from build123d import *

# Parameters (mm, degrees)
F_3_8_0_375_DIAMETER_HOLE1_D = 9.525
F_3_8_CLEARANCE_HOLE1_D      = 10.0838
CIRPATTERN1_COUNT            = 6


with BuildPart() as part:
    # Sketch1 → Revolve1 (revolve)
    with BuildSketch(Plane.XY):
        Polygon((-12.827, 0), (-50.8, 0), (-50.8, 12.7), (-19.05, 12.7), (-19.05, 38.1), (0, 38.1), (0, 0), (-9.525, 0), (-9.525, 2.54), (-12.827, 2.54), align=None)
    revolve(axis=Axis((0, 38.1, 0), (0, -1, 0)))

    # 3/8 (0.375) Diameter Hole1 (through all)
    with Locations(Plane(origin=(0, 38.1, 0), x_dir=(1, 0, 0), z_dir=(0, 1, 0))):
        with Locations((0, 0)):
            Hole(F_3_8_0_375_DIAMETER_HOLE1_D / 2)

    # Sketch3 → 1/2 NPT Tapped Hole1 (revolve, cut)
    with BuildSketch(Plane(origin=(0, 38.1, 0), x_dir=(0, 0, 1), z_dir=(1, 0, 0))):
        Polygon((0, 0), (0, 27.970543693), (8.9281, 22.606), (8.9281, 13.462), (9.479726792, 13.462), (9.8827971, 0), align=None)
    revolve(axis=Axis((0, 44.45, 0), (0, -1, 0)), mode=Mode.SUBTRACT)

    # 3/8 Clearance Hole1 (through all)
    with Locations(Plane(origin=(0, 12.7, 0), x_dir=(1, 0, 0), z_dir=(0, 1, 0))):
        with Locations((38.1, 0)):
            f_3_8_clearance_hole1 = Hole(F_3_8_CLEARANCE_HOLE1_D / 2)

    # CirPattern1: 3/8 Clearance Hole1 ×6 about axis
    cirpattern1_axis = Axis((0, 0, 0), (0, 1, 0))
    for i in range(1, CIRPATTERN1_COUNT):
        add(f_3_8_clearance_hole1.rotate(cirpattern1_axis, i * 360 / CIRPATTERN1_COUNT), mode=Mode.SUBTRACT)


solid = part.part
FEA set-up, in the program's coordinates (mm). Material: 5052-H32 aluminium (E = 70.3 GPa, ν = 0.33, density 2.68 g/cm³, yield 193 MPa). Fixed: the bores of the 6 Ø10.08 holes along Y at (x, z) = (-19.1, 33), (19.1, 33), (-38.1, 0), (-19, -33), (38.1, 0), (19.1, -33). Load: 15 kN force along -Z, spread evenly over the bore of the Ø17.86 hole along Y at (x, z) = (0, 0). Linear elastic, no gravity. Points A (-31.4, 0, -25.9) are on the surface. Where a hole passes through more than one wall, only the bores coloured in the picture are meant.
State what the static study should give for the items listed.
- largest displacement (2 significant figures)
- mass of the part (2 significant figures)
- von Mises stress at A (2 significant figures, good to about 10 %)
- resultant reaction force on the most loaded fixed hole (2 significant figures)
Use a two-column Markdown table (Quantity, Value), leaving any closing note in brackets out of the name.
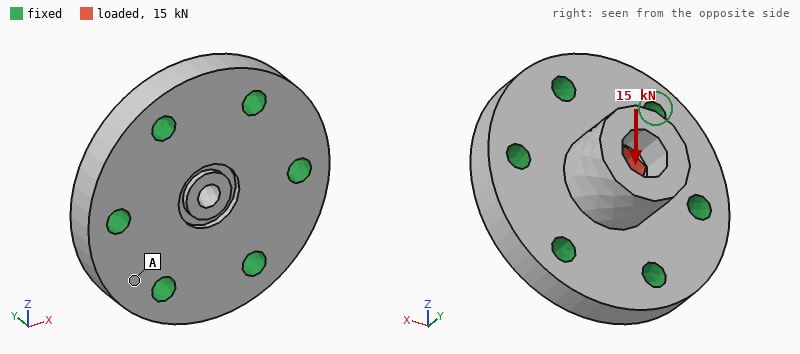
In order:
| Quantity | Value |
|---|---|
| largest displacement | 24 µm |
| mass of the part | 320 g |
| von Mises stress at A | 4.7 MPa |
| resultant reaction force on the most loaded fixed hole | 4.0 kN |
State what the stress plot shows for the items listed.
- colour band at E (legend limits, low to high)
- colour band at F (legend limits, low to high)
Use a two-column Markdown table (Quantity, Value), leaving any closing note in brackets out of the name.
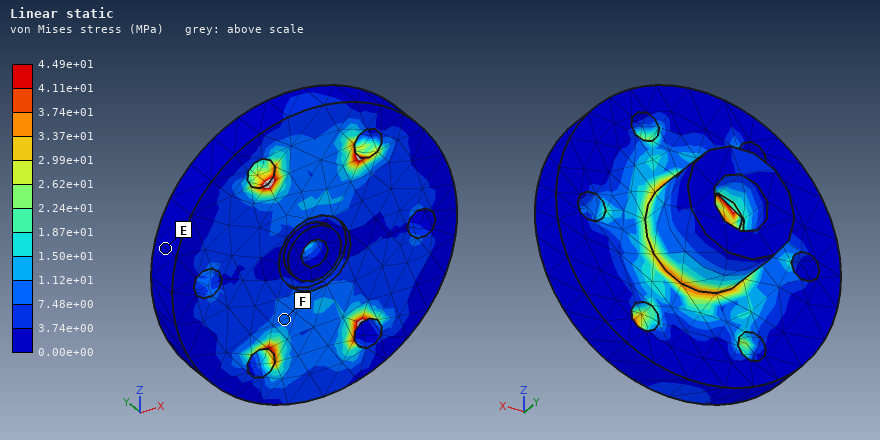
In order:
| Quantity | Value |
|---|---|
| colour band at E | 0.00e+00 to 3.74e+00 MPa |
| colour band at F | 7.48e+00 to 1.12e+01 MPa |
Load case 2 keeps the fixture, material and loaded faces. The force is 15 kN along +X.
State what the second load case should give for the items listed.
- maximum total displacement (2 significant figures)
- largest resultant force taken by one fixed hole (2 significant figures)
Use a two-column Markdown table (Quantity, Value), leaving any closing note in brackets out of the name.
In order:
| Quantity | Value |
|---|---|
| maximum total displacement | 24 µm |
| largest resultant force taken by one fixed hole | 4.5 kN |
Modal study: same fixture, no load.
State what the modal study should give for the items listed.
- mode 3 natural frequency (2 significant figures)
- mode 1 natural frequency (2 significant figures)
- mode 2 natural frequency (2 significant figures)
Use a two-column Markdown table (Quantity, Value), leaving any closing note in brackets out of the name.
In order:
| Quantity | Value |
|---|---|
| mode 3 natural frequency | 14 kHz |
| mode 1 natural frequency | 14 kHz |
| mode 2 natural frequency | 14 kHz |
